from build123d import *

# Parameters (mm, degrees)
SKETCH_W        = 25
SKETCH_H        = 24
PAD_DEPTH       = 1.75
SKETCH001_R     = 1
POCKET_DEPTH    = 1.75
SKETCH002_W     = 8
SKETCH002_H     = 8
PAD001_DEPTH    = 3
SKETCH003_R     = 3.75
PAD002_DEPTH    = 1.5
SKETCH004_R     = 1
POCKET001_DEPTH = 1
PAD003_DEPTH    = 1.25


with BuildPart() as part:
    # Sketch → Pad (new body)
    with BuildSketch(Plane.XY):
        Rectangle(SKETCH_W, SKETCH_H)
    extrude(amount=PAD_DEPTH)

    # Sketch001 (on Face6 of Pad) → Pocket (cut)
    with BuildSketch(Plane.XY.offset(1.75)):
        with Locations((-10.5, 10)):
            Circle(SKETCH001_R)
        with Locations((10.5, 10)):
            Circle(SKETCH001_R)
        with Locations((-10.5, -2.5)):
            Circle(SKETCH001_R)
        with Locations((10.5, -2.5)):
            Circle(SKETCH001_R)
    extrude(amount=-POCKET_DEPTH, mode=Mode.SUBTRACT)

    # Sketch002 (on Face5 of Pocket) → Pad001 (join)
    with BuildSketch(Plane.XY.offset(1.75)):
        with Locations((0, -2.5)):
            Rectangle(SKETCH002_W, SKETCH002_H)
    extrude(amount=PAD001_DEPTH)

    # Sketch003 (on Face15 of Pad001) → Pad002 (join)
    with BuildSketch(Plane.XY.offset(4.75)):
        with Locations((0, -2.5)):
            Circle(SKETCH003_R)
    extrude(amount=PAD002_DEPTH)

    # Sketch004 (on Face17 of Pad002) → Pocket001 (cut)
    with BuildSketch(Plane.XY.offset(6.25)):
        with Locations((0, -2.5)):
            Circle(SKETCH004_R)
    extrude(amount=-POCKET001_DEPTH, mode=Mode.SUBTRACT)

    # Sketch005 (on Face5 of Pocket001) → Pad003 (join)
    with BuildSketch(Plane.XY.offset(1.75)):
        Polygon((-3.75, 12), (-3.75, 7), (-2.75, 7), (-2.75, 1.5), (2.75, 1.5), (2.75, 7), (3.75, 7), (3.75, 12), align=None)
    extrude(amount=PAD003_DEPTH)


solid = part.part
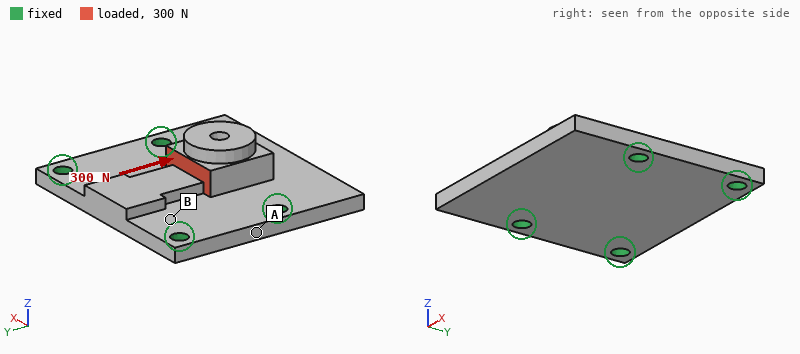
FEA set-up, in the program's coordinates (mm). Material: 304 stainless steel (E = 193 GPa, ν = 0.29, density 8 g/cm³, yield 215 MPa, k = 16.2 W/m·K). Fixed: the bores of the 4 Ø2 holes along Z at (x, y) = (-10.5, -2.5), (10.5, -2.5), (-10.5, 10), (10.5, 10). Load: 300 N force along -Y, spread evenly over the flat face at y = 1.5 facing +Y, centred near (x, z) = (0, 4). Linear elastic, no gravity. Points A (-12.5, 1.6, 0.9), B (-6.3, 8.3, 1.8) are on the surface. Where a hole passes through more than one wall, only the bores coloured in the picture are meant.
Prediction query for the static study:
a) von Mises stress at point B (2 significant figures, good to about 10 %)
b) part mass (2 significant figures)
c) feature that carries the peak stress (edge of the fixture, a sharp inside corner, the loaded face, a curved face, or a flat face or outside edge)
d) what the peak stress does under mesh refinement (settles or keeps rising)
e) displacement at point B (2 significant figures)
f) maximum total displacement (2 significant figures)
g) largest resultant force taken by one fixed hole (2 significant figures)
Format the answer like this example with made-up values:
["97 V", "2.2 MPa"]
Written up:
["13 MPa", "11 g", "edge of the fixture", "keeps rising", "0.93 µm", "5.4 µm", "98 N"]
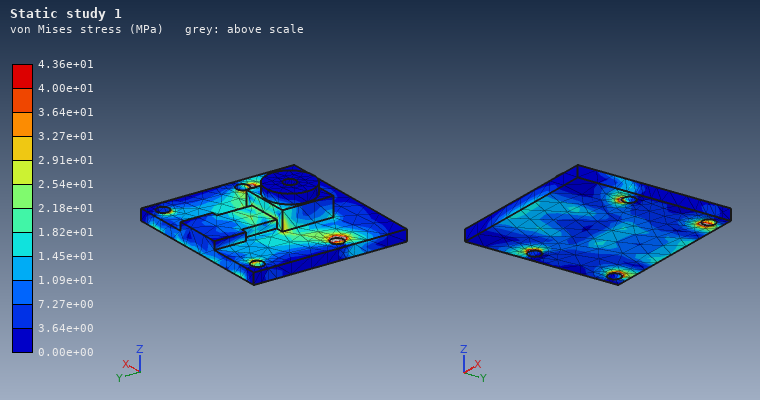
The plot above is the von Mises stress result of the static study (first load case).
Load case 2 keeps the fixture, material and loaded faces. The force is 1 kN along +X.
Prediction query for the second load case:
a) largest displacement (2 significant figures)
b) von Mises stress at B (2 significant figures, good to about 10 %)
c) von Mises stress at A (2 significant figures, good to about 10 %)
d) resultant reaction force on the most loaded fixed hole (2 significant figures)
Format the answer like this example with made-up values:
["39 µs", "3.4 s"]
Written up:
["7.8 µm", "28 MPa", "13 MPa", "360 N"]
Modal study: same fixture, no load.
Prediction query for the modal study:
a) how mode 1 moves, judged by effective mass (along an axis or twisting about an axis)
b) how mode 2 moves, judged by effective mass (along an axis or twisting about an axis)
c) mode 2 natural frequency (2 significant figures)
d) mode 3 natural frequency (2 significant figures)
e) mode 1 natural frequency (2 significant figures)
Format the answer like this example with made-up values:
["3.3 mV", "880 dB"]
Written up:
["along Z", "along Z", "18 kHz", "22 kHz", "13 kHz"]
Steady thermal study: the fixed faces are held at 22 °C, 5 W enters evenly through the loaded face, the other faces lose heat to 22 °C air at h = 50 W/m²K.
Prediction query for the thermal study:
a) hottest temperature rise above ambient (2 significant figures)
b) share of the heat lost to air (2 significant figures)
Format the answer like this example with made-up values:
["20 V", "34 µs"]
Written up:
["72 K", "28 %"]
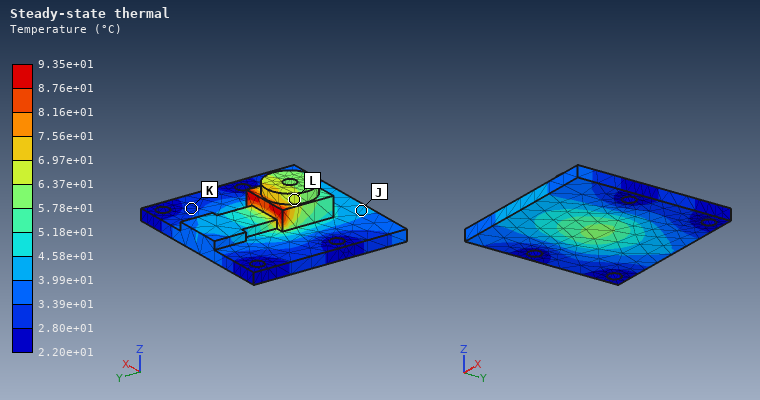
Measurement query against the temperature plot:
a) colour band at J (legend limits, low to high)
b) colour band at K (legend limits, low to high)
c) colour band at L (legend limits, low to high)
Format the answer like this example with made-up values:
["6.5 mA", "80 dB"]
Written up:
["3.99e+01 to 4.58e+01 °C", "2.80e+01 to 3.39e+01 °C", "6.37e+01 to 6.97e+01 °C"]
